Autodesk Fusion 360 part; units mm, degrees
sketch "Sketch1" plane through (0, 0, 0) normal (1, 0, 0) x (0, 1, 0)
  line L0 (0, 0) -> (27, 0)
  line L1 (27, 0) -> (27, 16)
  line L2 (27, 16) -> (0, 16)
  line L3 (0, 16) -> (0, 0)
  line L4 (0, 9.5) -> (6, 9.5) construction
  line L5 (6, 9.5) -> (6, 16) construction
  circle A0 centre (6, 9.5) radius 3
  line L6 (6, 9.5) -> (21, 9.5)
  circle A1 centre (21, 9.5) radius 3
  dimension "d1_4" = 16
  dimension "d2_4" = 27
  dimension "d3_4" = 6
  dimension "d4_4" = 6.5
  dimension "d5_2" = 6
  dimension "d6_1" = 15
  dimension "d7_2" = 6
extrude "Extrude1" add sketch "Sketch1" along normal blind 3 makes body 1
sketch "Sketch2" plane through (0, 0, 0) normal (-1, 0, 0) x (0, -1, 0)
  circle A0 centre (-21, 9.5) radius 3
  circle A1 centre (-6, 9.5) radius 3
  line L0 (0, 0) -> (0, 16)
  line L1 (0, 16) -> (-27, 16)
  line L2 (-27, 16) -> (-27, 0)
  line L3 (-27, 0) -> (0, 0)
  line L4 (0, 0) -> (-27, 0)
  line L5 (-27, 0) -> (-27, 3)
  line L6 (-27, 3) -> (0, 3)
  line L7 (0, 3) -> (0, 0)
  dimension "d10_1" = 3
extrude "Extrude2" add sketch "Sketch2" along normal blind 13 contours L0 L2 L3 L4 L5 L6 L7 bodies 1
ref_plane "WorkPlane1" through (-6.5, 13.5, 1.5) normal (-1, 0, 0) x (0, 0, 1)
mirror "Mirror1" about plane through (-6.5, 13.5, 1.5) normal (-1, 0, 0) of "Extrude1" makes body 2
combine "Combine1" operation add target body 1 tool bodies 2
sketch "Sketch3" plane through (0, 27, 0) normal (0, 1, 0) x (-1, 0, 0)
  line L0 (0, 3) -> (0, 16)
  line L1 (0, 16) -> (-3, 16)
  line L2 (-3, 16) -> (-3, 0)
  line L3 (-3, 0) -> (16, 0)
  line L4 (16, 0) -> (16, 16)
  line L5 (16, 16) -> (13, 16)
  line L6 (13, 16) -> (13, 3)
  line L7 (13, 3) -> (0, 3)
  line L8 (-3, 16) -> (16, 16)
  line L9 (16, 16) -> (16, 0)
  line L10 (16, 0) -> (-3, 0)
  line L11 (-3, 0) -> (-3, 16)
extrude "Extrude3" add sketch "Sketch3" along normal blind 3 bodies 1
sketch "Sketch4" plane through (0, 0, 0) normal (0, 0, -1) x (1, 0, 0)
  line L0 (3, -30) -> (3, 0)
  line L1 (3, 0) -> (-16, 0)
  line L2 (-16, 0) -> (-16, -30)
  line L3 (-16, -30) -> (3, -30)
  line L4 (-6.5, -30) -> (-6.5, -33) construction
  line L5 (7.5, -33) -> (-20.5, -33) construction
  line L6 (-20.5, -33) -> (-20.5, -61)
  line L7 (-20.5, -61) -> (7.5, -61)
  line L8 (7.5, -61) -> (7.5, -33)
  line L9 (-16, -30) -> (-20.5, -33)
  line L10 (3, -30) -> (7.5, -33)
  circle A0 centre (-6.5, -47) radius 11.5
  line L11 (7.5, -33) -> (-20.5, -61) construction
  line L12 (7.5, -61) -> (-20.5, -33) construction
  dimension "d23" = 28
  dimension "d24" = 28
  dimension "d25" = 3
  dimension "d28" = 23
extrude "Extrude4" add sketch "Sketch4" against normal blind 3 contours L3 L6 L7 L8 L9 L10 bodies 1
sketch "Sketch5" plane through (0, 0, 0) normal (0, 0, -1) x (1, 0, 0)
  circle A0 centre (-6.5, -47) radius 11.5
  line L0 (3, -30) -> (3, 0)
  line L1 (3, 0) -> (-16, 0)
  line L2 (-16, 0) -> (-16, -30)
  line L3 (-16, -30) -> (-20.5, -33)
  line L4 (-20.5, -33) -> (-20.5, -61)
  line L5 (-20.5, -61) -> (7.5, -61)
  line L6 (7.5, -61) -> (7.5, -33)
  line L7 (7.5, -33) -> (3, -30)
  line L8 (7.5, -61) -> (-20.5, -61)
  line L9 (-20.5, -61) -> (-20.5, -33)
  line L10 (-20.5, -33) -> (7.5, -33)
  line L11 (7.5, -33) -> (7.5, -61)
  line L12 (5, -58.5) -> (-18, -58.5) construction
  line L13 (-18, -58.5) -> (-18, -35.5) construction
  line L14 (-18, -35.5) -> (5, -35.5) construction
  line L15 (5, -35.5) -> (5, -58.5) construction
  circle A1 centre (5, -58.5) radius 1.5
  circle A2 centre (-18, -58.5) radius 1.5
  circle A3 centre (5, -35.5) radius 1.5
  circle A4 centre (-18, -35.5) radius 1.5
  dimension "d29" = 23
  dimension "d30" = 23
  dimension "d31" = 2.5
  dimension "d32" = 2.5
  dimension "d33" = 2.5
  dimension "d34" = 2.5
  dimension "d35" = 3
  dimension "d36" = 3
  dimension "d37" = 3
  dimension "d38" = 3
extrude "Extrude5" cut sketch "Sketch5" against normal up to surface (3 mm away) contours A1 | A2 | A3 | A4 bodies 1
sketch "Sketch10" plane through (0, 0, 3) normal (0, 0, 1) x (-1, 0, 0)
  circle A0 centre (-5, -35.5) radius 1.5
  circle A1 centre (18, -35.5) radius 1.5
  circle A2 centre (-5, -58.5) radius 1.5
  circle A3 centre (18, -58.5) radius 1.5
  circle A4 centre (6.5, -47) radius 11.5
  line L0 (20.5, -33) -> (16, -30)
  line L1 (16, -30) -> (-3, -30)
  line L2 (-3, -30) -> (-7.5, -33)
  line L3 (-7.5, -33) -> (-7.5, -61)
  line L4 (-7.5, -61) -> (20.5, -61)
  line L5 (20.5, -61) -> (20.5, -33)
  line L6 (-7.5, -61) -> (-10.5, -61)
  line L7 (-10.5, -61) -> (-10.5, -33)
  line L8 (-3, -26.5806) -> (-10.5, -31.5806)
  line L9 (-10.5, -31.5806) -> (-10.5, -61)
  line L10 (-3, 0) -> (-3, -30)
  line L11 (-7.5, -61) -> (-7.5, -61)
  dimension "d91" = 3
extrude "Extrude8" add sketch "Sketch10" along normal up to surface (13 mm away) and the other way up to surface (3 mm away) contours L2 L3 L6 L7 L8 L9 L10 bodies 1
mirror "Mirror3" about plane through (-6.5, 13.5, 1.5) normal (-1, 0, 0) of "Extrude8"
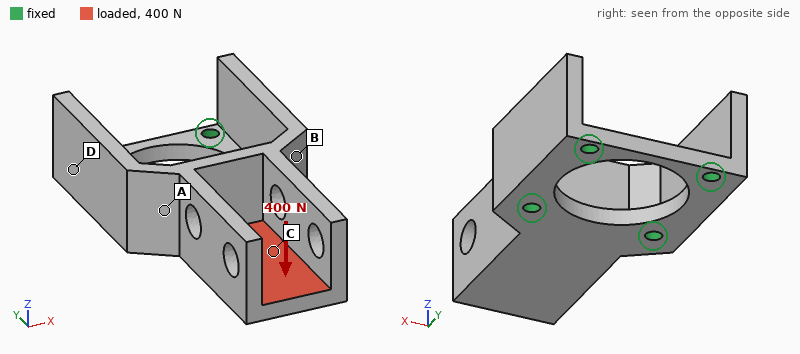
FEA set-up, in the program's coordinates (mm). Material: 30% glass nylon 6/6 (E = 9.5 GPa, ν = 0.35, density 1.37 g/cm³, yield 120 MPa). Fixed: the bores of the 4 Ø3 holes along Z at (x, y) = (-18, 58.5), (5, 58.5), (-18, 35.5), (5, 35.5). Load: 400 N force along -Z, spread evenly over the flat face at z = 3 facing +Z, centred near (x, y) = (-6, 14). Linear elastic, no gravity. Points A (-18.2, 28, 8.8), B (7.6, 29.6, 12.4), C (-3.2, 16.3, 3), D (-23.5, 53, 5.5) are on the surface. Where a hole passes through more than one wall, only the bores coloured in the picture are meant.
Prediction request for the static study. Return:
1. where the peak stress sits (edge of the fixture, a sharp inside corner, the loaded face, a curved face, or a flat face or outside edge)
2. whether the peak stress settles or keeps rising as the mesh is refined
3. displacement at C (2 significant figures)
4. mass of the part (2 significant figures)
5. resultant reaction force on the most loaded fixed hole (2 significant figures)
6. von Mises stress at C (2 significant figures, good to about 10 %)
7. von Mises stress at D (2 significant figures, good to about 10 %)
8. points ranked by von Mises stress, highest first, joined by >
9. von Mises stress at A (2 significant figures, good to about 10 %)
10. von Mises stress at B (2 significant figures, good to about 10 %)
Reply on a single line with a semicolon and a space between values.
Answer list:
edge of the fixture; keeps rising; 0.30 mm; 12 g; 370 N; 5.5 MPa; 10 MPa; A > B > D > C; 40 MPa; 33 MPa
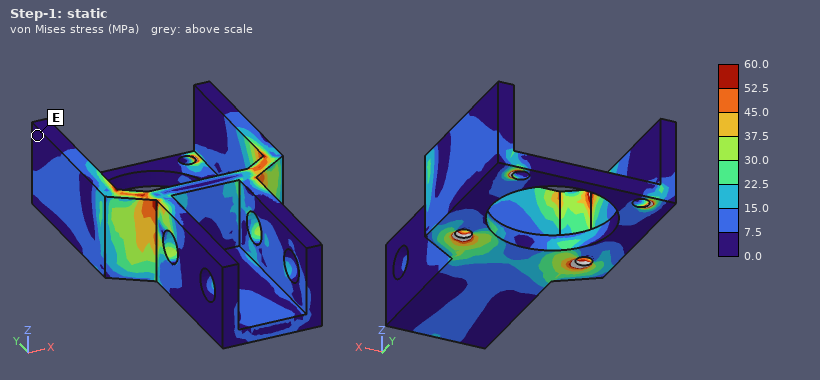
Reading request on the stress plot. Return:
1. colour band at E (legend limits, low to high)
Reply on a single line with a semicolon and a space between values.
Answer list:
0.0 to 7.5 MPa
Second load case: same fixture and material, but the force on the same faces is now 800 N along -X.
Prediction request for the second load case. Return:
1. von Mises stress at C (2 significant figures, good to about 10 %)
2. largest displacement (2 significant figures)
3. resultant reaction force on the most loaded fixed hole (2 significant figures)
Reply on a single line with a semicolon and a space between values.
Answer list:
28 MPa; 0.35 mm; 770 N
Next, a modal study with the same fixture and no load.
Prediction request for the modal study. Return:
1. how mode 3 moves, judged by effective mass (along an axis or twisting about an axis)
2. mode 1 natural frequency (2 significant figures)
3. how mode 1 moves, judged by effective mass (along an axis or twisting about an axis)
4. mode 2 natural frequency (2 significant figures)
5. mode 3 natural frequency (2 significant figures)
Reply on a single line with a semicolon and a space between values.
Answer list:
along X; 2200 Hz; along Z; 3300 Hz; 5100 Hz
